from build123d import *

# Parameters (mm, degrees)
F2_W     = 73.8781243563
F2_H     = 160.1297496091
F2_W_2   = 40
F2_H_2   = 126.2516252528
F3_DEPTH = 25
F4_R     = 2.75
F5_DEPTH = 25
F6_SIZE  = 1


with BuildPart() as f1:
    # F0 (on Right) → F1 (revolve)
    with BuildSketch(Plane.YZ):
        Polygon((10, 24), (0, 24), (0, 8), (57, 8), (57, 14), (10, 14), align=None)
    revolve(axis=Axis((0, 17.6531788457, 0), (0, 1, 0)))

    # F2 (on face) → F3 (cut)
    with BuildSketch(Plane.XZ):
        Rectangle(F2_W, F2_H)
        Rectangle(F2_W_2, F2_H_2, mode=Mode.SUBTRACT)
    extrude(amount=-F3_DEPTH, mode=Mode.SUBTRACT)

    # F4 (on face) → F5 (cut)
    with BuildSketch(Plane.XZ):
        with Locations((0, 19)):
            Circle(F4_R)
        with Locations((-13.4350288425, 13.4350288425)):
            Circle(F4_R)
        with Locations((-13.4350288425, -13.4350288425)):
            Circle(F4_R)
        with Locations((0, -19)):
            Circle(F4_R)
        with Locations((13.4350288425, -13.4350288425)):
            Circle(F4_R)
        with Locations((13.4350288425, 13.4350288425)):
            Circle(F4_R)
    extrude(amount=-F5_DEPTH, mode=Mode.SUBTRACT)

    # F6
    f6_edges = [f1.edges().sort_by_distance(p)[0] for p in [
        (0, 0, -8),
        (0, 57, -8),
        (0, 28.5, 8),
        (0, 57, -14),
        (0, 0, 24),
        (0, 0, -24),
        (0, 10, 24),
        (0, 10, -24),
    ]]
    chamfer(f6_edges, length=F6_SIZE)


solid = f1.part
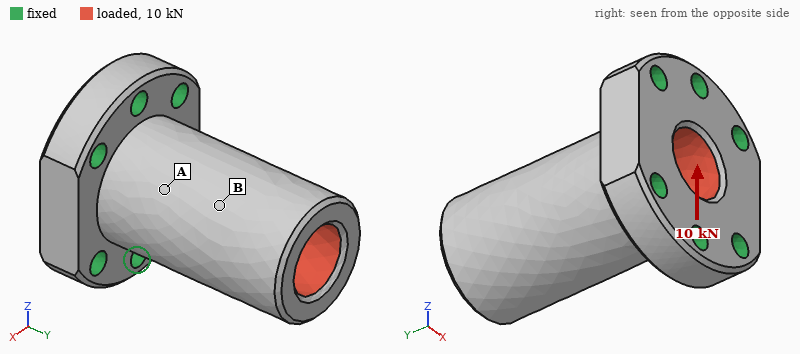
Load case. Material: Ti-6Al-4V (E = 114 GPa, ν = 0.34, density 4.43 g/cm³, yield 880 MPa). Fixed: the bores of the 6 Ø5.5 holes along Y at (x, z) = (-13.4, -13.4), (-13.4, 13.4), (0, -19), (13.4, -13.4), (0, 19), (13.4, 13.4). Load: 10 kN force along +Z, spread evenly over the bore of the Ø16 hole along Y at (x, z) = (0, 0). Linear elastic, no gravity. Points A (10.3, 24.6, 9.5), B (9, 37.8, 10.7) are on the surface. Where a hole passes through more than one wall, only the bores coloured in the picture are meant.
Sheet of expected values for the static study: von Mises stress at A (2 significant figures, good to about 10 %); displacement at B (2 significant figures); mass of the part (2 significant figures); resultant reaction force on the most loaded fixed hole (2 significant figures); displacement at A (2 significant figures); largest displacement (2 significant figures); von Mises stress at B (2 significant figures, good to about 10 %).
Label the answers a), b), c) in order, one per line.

a) 39 MPa
b) 45 µm
c) 140 g
d) 4.2 kN
e) 24 µm
f) 73 µm
g) 19 MPa
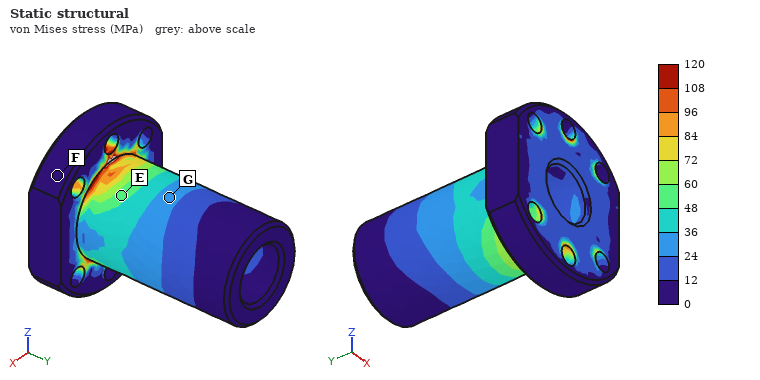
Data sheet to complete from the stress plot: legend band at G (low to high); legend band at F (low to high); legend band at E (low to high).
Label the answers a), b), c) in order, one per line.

a) 24 to 36 MPa
b) 0 to 12 MPa
c) 48 to 60 MPa
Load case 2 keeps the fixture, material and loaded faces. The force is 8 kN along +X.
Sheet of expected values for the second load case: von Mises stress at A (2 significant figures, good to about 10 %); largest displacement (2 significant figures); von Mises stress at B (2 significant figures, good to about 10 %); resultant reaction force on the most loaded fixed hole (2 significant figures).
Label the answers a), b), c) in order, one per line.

a) 32 MPa
b) 68 µm
c) 16 MPa
d) 4.0 kN
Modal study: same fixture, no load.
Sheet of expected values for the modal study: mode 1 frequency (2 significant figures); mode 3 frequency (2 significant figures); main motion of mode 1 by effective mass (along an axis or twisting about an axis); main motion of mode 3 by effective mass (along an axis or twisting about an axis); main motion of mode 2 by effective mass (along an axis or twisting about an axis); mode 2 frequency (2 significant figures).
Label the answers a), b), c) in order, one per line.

a) 6400 Hz
b) 15 kHz
c) along X
d) twisting about Y
e) along Z
f) 6900 Hz
